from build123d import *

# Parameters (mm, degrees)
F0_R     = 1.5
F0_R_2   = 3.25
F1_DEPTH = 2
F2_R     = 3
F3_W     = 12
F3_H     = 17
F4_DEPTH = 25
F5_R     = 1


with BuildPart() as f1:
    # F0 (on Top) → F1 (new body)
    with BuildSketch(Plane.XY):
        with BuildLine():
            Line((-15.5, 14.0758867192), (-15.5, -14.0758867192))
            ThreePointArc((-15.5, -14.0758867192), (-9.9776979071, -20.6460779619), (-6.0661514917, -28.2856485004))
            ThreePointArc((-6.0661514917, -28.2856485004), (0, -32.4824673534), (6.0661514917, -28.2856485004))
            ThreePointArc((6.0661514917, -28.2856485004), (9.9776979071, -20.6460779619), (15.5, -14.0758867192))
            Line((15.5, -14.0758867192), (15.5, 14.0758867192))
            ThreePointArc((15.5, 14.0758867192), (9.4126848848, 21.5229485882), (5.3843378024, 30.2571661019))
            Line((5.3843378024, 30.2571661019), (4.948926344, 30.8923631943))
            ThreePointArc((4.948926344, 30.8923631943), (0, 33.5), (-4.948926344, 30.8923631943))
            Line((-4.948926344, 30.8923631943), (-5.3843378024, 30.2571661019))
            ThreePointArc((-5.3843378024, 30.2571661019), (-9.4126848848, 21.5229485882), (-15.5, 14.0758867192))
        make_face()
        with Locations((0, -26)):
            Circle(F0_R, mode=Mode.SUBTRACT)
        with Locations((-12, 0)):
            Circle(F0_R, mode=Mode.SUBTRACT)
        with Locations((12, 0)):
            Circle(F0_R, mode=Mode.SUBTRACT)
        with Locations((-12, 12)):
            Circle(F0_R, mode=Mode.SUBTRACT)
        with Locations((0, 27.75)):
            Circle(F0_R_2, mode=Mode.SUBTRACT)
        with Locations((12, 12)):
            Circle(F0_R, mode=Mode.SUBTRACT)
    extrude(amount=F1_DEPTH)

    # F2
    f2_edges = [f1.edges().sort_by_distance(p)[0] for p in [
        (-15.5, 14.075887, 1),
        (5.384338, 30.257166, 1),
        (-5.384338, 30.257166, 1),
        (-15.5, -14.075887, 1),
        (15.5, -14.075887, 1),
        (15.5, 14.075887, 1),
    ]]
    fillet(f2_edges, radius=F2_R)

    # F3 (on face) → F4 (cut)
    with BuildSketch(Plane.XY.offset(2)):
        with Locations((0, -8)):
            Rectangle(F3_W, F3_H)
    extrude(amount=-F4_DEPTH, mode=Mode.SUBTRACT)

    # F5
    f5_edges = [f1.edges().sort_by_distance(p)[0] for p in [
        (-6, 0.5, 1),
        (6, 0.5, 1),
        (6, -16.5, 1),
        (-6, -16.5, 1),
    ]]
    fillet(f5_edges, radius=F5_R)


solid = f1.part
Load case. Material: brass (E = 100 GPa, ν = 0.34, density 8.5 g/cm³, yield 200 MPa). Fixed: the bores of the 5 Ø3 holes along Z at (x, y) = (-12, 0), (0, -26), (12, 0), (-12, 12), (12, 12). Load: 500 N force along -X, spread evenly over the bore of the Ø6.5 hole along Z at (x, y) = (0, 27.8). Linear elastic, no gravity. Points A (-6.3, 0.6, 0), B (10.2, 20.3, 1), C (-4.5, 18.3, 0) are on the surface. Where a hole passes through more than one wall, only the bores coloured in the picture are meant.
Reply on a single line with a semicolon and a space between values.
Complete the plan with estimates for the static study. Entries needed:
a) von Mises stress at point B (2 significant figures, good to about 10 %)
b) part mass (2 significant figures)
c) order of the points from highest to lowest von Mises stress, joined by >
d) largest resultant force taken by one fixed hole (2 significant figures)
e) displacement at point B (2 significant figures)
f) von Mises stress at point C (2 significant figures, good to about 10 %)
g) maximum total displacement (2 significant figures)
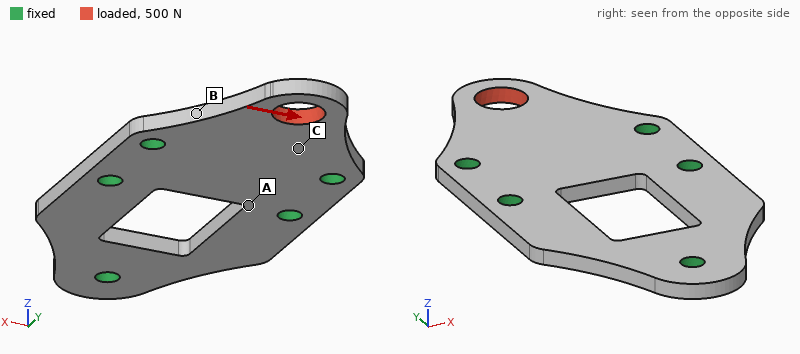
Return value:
43 MPa; 21 g; B > C > A; 380 N; 3.0 µm; 15 MPa; 16 µm
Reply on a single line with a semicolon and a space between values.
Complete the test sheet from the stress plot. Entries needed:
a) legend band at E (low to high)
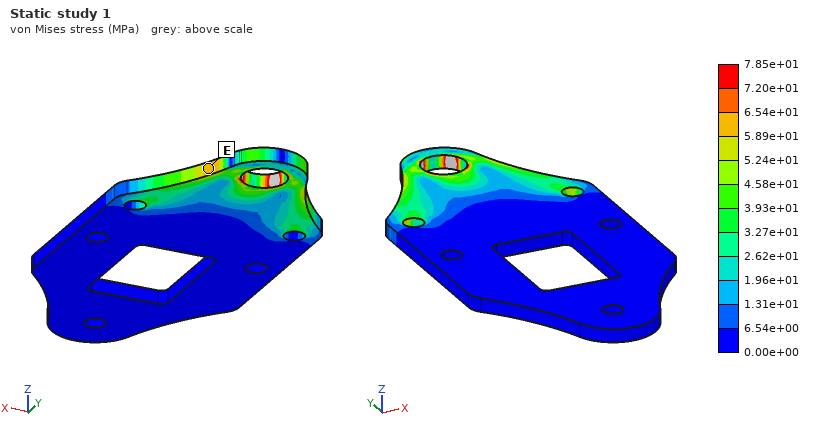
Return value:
5.89e+01 to 6.54e+01 MPa
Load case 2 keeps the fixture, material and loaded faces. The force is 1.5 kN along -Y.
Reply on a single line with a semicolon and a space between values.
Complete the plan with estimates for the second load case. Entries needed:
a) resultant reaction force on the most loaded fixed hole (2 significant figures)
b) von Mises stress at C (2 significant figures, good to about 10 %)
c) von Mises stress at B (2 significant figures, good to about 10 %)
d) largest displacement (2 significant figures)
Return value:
580 N; 34 MPa; 50 MPa; 16 µm
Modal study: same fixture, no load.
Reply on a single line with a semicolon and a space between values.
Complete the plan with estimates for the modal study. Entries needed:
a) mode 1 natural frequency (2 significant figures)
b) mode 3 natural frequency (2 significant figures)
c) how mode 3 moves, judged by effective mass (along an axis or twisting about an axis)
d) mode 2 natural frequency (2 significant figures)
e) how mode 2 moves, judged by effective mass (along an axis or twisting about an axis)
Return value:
3600 Hz; 8500 Hz; along Z; 8100 Hz; twisting about Y
